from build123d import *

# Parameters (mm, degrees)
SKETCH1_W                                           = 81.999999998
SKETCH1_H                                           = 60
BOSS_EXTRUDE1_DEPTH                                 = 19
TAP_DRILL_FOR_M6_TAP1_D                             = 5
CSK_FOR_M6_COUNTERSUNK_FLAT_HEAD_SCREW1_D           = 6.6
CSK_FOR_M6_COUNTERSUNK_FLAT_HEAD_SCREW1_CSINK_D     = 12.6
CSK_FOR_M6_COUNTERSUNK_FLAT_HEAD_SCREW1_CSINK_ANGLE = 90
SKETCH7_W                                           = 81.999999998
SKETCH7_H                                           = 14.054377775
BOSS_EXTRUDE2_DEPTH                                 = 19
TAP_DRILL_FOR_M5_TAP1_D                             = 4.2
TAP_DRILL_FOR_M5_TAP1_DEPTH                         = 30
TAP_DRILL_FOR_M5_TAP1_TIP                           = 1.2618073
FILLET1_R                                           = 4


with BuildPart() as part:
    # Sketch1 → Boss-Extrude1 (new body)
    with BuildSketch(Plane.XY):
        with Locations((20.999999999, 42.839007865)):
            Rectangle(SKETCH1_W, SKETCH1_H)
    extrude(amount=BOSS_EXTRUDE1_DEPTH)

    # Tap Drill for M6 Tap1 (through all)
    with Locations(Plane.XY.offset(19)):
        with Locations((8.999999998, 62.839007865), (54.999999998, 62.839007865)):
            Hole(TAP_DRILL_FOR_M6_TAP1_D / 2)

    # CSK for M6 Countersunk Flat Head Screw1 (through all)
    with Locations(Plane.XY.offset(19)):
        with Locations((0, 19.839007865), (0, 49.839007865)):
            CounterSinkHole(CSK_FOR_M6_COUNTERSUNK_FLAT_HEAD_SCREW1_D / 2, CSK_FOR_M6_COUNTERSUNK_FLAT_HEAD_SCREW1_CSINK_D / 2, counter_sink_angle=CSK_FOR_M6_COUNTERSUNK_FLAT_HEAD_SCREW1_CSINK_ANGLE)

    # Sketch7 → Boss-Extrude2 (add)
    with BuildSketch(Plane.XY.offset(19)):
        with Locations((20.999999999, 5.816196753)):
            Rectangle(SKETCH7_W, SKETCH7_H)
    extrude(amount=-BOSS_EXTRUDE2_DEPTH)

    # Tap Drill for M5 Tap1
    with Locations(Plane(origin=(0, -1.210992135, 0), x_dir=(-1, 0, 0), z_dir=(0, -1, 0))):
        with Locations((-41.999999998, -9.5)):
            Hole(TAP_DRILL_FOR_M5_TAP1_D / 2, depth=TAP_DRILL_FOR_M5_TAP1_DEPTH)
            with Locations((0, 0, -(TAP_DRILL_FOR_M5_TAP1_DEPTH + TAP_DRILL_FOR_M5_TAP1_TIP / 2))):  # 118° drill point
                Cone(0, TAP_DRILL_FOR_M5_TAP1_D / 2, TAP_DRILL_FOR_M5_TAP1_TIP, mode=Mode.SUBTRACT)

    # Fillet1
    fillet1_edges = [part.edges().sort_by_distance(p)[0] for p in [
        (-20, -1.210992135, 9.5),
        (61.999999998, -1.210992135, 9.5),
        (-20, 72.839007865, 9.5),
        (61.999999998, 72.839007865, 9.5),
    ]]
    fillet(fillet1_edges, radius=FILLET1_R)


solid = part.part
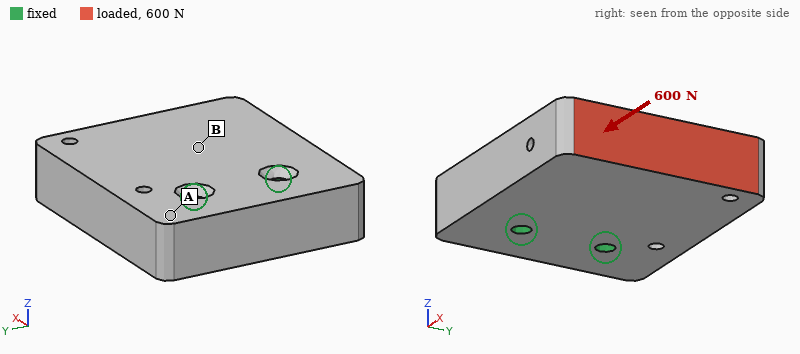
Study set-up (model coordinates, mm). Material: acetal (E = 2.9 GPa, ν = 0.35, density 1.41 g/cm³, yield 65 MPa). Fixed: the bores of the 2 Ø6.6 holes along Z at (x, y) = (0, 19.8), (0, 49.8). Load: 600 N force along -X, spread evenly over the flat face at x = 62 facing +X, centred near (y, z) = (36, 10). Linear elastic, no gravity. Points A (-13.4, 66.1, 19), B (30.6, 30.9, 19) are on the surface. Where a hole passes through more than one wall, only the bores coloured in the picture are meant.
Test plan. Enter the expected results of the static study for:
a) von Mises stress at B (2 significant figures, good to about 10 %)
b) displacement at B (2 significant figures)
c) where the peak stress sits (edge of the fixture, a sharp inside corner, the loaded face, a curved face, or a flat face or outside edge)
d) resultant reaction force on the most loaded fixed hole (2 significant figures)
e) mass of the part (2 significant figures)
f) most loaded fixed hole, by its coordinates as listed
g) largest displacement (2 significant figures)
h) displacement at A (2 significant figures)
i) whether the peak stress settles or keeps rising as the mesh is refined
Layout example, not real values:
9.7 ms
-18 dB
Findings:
0.55 MPa
7.2 µm
edge of the fixture
320 N
160 g
(0, 49.8)
14 µm
4.4 µm
keeps rising
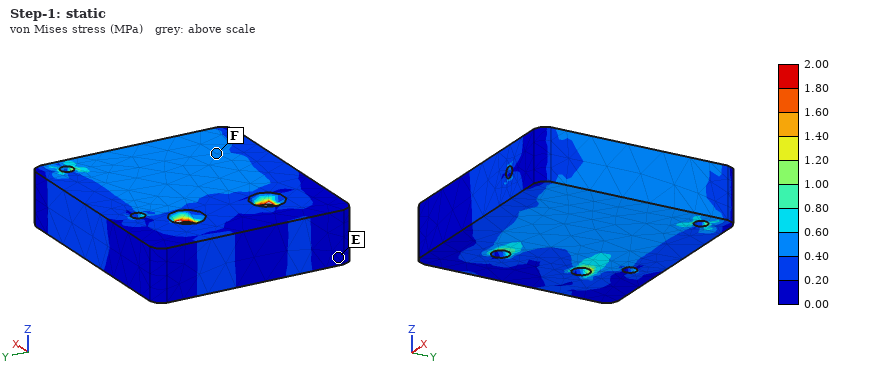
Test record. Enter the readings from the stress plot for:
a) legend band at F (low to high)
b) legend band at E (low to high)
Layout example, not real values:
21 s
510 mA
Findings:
0.40 to 0.60 MPa
0.00 to 0.20 MPa
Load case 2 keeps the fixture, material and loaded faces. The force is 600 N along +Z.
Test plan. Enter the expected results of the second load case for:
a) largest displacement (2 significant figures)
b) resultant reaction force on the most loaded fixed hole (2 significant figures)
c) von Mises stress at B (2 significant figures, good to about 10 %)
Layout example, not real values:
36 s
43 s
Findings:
0.57 mm
310 N
4.1 MPa
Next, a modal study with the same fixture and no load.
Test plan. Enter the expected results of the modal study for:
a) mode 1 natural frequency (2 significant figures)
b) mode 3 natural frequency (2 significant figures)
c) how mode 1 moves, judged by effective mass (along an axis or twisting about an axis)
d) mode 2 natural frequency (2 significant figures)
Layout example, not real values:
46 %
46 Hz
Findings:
910 Hz
1800 Hz
along Z
1700 Hz
